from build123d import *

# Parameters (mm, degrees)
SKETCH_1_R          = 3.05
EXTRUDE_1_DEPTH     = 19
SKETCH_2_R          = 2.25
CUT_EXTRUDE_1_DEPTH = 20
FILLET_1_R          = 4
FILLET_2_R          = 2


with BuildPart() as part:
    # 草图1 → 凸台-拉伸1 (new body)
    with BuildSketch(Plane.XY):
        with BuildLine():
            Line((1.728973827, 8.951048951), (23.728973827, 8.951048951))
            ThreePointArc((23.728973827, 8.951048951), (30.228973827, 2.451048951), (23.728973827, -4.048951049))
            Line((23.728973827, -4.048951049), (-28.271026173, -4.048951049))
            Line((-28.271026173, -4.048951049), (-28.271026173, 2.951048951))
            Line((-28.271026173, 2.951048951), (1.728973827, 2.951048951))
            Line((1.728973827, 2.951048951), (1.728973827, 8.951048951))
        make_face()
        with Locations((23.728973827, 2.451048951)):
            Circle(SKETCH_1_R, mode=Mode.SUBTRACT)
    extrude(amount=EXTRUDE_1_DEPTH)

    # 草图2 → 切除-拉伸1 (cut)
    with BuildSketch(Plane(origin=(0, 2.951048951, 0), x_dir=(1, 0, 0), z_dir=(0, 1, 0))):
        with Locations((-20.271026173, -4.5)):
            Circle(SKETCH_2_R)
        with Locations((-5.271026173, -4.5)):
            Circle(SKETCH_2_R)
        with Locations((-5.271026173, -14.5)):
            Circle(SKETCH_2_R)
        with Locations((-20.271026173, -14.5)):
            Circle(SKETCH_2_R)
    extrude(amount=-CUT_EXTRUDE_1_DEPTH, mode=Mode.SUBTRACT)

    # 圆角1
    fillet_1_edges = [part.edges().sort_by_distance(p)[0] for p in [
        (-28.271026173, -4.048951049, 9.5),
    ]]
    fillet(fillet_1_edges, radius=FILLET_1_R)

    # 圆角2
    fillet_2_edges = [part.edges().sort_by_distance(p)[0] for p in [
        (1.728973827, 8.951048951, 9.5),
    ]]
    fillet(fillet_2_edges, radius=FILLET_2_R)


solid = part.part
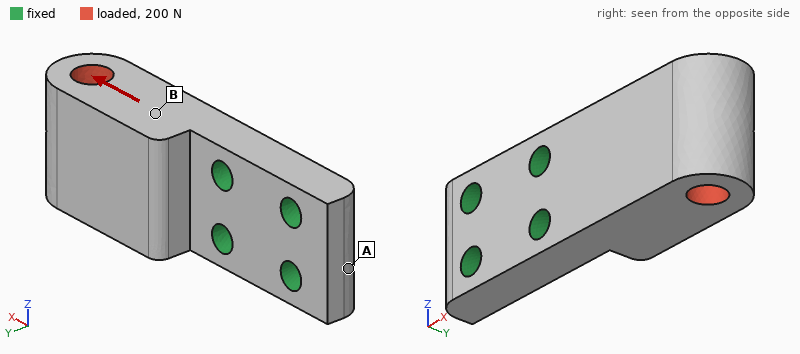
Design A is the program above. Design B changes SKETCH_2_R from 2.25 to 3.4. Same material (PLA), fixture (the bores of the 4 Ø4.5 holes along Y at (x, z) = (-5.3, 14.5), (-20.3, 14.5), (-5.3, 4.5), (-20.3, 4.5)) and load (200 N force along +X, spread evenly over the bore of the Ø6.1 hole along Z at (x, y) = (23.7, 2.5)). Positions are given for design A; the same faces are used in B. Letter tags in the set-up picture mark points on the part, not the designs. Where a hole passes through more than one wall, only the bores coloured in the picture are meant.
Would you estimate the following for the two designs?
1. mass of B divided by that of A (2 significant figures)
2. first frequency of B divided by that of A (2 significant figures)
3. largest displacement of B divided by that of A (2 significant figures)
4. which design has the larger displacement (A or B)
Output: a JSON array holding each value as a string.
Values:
["0.94", "1.1", "0.81", "A"]
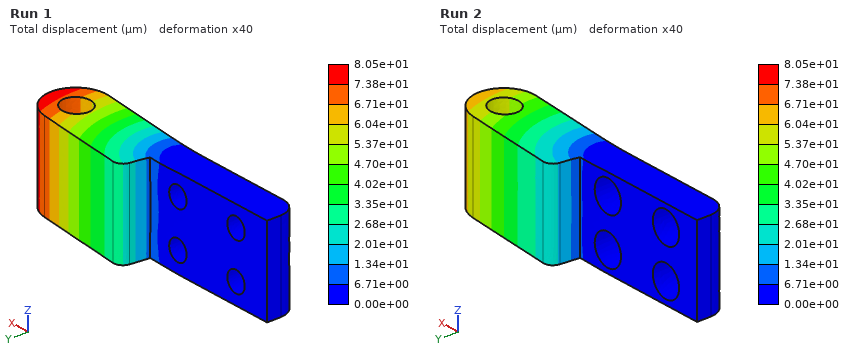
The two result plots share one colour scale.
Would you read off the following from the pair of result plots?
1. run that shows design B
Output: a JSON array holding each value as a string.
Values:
["Run 2"]
